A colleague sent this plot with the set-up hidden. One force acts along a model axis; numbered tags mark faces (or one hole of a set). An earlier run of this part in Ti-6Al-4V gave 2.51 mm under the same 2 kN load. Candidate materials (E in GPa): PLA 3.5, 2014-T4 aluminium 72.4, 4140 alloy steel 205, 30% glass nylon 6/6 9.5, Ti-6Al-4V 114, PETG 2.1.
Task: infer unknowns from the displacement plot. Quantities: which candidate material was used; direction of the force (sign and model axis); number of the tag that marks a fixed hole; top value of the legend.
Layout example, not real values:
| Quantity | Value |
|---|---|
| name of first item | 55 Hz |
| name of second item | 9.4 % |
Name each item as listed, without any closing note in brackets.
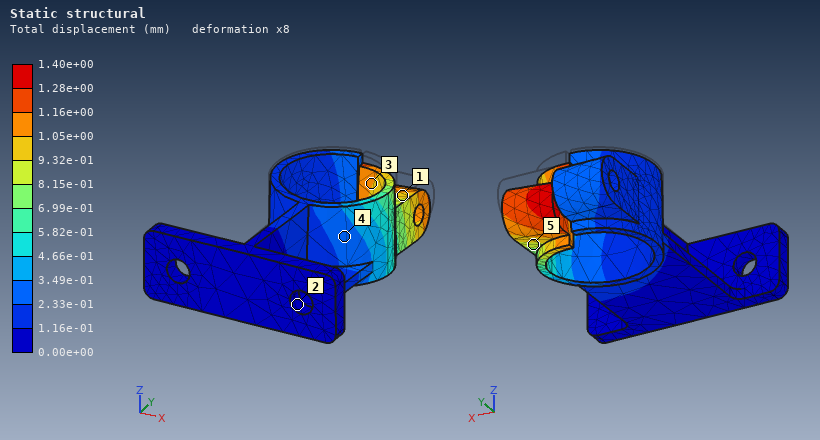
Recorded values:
| Quantity | Value |
|---|---|
| which candidate material was used | 4140 alloy steel |
| direction of the force | -Z |
| number of the tag that marks a fixed hole | 2 |
| top value of the legend | 1.40e+00 mm |
